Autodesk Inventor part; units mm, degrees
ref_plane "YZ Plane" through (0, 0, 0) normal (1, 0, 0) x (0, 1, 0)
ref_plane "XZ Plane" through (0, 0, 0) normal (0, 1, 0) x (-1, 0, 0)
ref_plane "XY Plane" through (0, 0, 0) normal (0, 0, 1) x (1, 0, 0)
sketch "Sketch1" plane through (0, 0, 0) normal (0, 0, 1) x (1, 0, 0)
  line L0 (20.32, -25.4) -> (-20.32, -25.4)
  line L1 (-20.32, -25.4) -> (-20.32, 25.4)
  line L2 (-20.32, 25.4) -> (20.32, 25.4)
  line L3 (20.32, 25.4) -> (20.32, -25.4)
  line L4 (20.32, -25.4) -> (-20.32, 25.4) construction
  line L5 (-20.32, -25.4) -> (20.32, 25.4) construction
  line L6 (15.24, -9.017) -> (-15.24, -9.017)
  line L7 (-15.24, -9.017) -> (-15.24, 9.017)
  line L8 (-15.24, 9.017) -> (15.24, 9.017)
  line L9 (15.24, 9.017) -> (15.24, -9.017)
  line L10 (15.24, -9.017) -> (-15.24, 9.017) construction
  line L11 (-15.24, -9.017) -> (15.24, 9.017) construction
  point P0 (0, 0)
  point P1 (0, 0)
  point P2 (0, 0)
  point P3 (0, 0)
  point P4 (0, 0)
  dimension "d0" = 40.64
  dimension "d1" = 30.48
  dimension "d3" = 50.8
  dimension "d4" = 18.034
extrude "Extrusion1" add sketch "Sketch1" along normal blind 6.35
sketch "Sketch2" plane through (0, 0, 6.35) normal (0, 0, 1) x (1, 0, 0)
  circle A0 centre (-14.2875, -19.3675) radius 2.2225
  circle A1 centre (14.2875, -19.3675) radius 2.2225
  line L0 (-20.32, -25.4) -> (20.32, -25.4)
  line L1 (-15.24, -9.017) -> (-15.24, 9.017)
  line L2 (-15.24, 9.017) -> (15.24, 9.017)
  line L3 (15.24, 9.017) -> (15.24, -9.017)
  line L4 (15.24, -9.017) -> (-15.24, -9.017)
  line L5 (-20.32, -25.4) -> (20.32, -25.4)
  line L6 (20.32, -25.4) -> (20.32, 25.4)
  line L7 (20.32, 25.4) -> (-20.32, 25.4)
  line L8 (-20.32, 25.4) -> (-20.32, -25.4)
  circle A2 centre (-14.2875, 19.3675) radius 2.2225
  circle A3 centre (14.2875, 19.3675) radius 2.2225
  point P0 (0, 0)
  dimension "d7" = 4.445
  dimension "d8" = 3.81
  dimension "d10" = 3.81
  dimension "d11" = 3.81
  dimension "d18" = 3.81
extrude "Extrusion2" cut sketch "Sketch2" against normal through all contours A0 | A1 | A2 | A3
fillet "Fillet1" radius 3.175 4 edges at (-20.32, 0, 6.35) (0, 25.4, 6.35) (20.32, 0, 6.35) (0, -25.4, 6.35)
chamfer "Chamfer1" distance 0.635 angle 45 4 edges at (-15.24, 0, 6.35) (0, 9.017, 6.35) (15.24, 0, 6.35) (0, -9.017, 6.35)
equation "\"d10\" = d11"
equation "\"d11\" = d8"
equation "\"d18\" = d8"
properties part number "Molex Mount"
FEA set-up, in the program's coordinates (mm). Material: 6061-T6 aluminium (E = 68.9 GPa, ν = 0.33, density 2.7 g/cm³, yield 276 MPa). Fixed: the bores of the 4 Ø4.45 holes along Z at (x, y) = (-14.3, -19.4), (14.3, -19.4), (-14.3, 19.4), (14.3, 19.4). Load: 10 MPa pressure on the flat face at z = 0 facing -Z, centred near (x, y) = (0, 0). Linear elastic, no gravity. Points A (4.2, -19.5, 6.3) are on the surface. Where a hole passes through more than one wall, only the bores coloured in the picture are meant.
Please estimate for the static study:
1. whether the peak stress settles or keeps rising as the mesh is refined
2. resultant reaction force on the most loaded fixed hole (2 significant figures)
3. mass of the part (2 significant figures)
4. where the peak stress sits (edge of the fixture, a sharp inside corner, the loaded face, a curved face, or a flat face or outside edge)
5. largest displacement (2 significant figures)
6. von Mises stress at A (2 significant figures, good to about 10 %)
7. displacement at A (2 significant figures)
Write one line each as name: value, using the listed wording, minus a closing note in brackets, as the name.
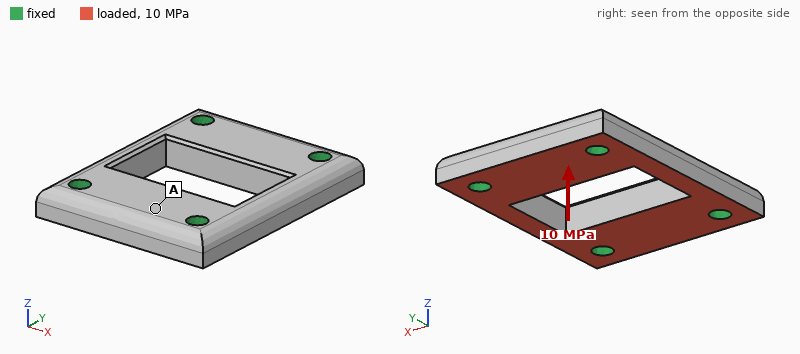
whether the peak stress settles or keeps rising as the mesh is refined: keeps rising
resultant reaction force on the most loaded fixed hole: 3.6 kN
mass of the part: 24 g
where the peak stress sits: edge of the fixture
largest displacement: 40 µm
von Mises stress at A: 38 MPa
displacement at A: 15 µm
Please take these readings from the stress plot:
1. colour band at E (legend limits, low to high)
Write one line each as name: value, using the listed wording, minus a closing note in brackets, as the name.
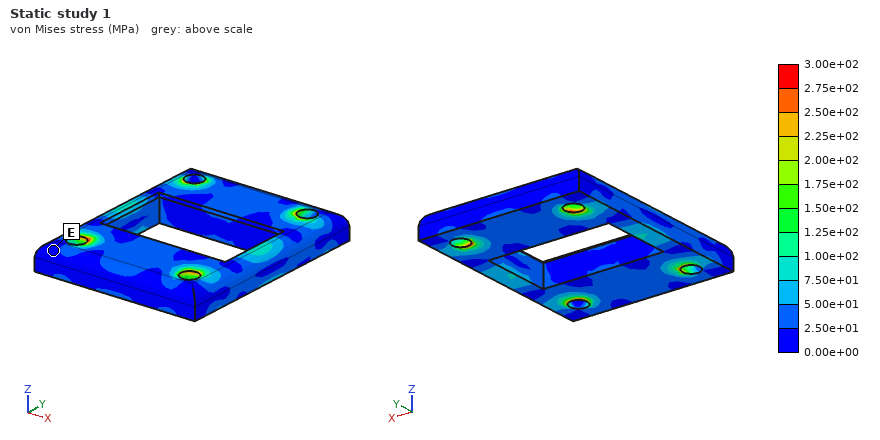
colour band at E: 0.00e+00 to 2.50e+01 MPa
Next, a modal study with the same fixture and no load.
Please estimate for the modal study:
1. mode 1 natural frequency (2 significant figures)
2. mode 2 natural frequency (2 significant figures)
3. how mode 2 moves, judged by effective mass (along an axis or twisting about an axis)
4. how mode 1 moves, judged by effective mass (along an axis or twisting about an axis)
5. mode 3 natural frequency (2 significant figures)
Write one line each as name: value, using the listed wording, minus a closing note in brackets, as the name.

mode 1 natural frequency: 24 kHz
mode 2 natural frequency: 25 kHz
how mode 2 moves, judged by effective mass: twisting about Y
how mode 1 moves, judged by effective mass: along Z
mode 3 natural frequency: 28 kHz
